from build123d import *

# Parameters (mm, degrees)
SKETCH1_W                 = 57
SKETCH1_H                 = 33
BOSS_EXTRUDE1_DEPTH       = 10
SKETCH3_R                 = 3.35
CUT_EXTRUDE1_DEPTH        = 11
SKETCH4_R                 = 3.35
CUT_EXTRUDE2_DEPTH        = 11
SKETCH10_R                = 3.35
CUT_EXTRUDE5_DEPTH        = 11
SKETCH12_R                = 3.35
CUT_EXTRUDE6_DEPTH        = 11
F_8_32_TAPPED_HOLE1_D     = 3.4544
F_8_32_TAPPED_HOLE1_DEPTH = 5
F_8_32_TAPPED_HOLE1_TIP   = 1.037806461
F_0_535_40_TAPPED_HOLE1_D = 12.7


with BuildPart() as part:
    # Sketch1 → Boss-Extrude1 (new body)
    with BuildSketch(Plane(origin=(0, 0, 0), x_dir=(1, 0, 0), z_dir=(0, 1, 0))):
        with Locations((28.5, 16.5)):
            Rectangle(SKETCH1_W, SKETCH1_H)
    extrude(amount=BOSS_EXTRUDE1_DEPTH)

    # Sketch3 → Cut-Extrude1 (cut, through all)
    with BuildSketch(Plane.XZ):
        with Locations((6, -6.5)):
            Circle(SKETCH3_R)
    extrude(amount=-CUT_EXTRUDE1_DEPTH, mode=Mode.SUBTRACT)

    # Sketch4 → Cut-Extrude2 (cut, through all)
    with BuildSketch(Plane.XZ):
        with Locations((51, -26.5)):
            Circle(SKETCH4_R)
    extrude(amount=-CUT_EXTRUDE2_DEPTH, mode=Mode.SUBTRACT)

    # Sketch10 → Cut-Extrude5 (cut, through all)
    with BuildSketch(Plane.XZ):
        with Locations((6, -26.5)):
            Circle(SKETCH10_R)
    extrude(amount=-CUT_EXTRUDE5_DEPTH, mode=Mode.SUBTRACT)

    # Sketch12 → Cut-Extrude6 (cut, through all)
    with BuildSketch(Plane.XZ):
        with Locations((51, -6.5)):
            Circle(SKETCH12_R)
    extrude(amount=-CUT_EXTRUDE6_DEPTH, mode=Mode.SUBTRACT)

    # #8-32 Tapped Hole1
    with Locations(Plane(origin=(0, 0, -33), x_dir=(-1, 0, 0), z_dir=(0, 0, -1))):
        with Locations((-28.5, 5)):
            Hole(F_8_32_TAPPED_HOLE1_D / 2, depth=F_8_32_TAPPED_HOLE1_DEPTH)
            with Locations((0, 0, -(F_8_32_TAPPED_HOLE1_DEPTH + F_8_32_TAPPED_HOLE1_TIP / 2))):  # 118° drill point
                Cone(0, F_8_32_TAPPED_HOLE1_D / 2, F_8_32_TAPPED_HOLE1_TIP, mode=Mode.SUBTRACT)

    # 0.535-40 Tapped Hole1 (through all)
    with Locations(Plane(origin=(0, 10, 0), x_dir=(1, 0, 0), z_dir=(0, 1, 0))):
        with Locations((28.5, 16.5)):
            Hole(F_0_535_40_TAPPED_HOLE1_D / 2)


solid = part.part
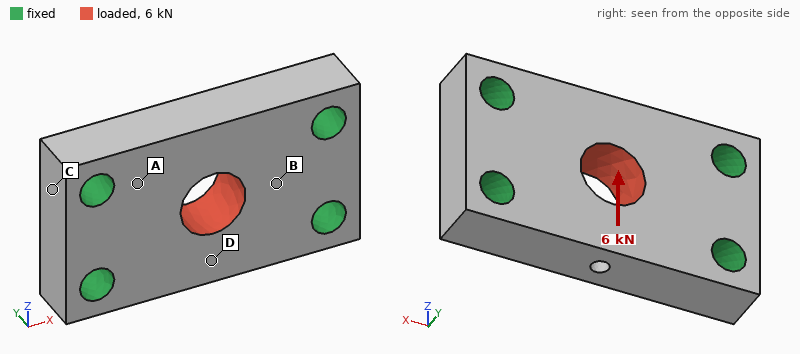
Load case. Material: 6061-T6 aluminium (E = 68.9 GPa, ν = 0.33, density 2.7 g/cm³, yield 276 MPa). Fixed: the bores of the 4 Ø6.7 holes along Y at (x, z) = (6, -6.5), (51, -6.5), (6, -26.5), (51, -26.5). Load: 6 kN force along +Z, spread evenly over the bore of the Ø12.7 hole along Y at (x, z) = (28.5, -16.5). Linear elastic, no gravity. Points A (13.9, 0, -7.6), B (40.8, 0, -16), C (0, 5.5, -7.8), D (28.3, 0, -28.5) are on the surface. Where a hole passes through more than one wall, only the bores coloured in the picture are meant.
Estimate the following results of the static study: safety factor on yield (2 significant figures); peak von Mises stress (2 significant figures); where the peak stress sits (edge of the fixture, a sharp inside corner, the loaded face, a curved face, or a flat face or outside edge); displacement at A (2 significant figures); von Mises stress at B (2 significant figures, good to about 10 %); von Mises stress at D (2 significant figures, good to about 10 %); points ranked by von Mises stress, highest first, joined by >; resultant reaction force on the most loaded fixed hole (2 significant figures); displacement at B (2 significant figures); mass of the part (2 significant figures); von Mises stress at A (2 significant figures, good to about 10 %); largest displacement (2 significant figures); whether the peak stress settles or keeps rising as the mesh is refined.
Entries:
5.3
52 MPa
a curved face
2.7 µm
24 MPa
11 MPa
B > A > D > C
1.9 kN
3.9 µm
43 g
18 MPa
9.4 µm
settles
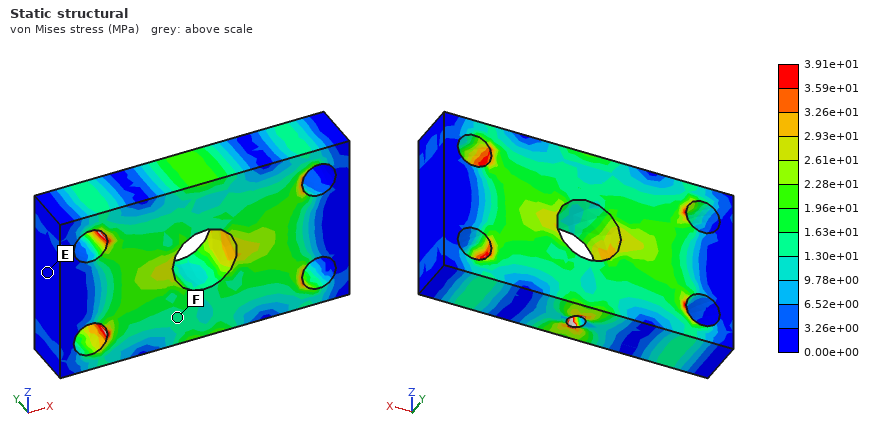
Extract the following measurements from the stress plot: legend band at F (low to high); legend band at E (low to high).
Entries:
1.30e+01 to 1.63e+01 MPa
0.00e+00 to 3.26e+00 MPa
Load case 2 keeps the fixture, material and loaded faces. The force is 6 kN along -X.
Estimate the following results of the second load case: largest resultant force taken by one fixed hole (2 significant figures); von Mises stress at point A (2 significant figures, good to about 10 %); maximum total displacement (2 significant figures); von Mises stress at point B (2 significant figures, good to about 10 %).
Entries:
1.6 kN
13 MPa
3.5 µm
12 MPa
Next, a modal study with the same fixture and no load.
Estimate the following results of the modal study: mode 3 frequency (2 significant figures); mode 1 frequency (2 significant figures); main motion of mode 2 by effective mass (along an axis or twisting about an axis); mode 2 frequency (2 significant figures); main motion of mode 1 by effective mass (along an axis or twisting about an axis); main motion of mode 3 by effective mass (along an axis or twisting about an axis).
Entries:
35 kHz
23 kHz
twisting about X
27 kHz
along Y
along Z
